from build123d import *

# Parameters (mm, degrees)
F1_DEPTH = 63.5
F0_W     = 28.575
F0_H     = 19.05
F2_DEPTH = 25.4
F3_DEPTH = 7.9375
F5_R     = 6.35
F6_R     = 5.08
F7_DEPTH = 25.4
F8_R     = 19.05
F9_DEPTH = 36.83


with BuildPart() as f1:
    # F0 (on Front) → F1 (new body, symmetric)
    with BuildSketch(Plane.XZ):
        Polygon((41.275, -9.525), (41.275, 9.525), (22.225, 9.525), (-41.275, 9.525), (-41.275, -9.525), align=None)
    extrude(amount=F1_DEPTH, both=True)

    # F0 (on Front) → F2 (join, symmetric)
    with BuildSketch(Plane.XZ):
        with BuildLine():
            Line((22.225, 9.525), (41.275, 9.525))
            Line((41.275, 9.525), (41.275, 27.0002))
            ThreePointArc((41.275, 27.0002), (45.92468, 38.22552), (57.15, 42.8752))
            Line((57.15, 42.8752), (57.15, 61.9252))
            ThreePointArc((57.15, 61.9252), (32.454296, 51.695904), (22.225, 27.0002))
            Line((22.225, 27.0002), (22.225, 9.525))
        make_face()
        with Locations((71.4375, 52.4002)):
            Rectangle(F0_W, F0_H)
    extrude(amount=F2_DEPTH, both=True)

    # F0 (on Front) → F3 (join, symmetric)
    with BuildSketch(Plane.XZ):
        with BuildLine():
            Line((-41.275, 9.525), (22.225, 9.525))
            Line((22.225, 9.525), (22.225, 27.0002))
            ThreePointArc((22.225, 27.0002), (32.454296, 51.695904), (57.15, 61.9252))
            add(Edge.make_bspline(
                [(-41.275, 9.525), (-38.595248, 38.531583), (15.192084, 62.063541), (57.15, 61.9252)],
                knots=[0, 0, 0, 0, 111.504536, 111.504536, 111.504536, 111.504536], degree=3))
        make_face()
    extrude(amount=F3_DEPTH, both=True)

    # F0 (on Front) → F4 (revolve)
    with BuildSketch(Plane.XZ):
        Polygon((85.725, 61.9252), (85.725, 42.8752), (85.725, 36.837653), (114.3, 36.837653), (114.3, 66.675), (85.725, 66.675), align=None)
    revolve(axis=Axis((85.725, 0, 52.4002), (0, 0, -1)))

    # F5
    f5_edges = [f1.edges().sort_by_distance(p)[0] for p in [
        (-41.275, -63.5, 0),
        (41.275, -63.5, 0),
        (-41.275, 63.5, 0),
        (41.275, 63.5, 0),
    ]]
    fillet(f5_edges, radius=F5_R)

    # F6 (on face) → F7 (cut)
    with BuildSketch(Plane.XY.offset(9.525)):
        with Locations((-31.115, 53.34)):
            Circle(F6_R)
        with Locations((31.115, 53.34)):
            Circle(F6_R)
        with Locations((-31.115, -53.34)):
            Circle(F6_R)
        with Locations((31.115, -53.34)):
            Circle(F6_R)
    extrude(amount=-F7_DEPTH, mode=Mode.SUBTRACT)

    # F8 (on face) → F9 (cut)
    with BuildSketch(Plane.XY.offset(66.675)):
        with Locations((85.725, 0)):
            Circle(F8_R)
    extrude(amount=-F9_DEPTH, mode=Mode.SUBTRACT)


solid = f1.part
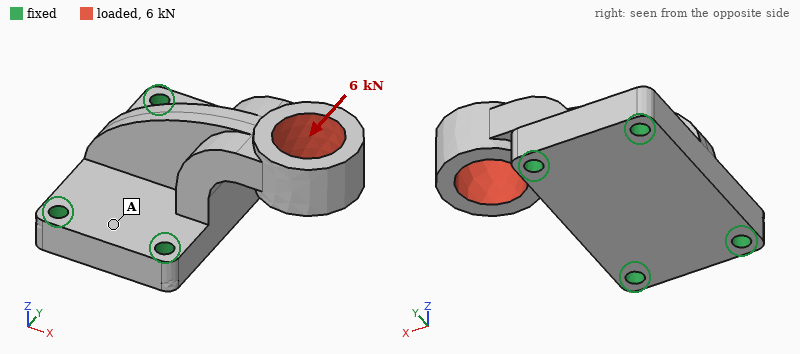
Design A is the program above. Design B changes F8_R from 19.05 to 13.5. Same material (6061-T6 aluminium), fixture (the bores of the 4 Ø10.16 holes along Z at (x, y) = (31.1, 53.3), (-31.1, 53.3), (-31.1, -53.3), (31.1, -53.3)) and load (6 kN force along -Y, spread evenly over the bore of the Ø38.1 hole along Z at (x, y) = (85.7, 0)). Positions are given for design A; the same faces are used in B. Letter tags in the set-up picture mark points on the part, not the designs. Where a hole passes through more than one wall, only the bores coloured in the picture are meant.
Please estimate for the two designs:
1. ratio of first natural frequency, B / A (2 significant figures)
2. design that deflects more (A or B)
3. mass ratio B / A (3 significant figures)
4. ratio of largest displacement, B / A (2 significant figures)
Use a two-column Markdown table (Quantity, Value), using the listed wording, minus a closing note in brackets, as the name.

| Quantity | Value |
|---|---|
| ratio of first natural frequency, B / A | 0.89 |
| design that deflects more | A |
| mass ratio B / A | 1.05 |
| ratio of largest displacement, B / A | 0.87 |
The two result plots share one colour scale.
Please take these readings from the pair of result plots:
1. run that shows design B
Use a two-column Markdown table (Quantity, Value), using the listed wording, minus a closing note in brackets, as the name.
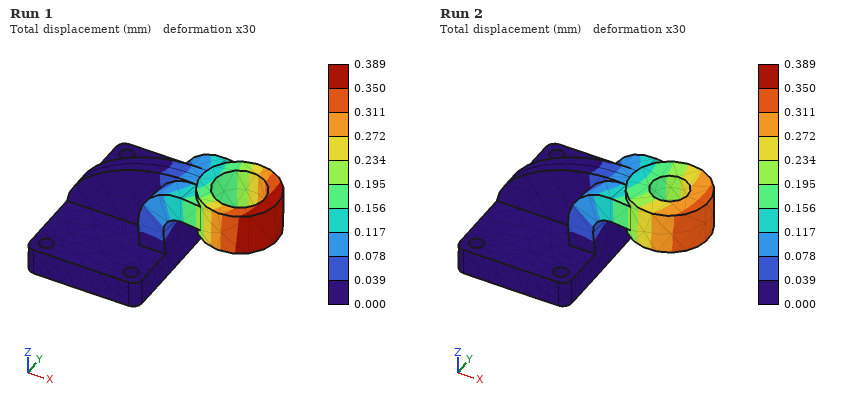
| Quantity | Value |
|---|---|
| run that shows design B | Run 2 |
